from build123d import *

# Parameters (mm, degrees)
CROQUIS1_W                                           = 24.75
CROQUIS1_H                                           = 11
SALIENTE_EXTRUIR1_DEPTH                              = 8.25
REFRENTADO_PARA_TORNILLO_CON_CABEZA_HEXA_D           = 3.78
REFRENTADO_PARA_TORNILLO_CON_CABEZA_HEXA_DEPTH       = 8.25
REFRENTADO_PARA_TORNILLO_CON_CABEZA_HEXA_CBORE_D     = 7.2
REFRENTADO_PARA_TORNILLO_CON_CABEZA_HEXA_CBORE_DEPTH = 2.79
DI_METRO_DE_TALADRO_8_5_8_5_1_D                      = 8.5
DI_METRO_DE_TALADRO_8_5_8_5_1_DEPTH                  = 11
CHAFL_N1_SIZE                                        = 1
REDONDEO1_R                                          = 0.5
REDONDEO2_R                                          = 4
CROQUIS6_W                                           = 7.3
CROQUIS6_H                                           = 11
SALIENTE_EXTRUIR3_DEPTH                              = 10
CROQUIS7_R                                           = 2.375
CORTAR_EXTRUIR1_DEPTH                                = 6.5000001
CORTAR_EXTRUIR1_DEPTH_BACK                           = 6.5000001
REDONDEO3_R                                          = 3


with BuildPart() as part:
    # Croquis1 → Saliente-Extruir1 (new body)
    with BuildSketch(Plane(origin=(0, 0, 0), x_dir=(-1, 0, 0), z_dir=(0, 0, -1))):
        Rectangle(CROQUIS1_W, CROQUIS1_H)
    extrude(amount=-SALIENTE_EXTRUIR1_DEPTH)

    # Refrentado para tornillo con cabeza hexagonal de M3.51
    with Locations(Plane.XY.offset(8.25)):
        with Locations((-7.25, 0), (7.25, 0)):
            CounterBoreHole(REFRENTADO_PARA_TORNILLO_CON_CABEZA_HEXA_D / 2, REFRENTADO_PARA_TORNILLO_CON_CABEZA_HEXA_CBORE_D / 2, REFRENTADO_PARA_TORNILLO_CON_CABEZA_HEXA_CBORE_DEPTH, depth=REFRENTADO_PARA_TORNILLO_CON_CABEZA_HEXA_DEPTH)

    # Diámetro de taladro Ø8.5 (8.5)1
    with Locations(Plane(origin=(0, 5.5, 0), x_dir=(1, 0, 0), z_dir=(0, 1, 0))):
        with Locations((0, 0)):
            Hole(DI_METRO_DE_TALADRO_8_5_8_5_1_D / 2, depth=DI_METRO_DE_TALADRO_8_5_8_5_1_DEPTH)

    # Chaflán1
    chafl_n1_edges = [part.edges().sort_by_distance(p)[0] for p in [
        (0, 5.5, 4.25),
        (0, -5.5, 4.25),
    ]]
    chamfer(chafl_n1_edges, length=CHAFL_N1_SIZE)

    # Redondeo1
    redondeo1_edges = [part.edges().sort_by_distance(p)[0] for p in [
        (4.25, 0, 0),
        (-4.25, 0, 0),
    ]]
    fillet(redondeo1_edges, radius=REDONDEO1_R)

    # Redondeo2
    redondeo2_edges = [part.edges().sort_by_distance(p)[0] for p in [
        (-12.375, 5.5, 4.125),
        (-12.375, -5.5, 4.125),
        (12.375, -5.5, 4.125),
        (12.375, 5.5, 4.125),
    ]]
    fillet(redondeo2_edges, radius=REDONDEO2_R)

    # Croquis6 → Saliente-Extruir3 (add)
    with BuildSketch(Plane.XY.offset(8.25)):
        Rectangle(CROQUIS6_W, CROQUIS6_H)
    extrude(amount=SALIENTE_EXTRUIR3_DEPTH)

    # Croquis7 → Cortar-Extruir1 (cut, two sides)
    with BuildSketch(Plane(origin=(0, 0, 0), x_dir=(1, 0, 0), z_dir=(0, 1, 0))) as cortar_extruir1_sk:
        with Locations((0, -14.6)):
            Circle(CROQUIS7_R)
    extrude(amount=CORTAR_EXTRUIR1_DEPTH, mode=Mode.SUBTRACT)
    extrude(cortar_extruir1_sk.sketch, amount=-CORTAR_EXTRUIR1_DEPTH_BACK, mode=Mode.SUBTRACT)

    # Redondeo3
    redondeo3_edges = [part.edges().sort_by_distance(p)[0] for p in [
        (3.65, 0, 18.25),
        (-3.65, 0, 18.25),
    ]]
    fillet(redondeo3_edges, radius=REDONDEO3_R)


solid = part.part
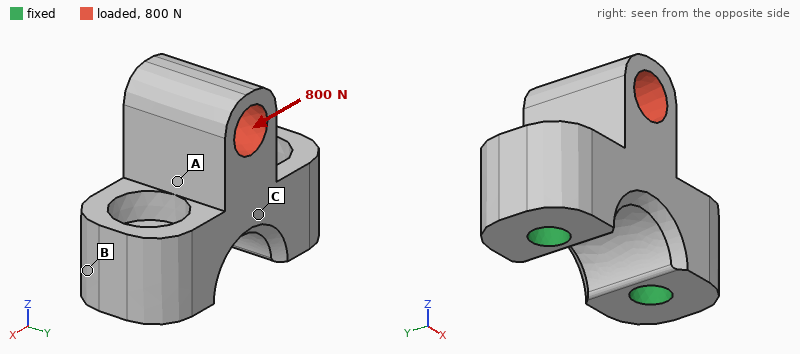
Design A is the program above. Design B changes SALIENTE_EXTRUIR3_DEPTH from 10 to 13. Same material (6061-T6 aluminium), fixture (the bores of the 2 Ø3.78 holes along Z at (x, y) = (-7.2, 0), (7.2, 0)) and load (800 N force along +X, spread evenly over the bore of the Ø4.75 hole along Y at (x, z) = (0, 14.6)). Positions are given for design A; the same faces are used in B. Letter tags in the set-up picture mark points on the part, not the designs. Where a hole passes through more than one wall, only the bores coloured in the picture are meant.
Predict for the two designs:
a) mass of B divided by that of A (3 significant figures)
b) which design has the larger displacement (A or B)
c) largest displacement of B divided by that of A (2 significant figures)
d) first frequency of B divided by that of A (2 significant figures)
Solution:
1.12
B
1.1
0.69
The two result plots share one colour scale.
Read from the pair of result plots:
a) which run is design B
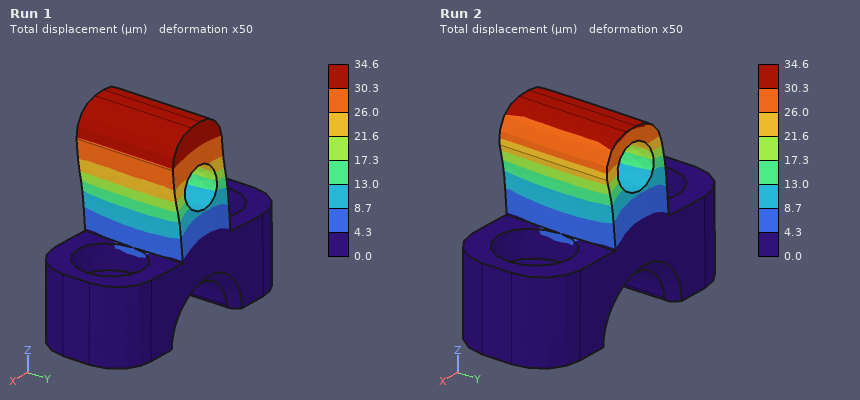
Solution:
Run 1
